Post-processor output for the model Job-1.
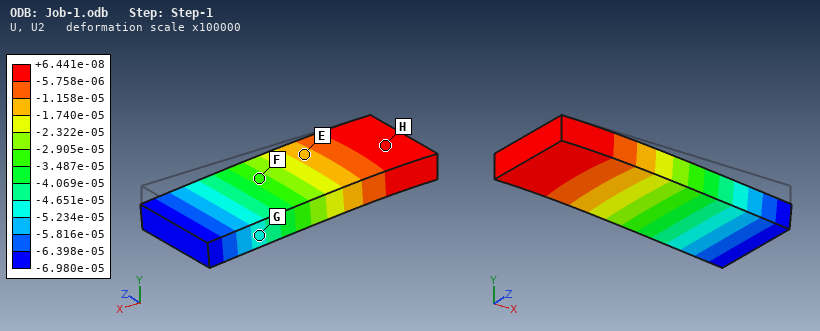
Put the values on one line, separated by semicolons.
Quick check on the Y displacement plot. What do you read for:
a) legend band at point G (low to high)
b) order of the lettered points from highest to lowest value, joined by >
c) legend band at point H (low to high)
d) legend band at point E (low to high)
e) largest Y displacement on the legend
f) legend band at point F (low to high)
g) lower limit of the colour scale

-5.234e-05 to -4.651e-05; H > E > F > G; -5.758e-06 to +6.441e-08; -1.740e-05 to -1.158e-05; +6.441e-08; -3.487e-05 to -2.905e-05; -6.980e-05
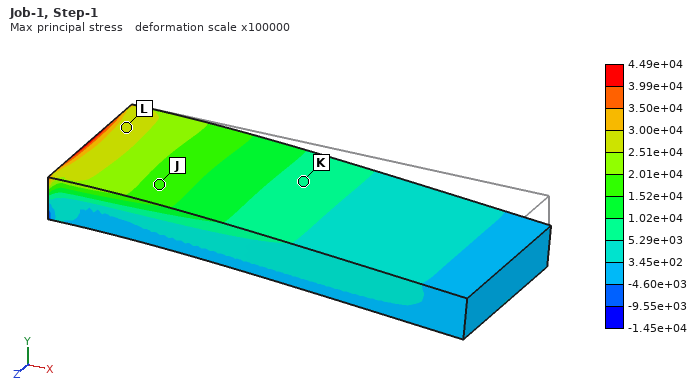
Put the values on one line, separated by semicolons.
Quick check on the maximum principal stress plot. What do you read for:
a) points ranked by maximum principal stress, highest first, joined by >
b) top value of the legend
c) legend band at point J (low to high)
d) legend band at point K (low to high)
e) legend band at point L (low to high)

L > J > K; 4.49e+04; 1.52e+04 to 2.01e+04; 5.29e+03 to 1.02e+04; 2.51e+04 to 3.00e+04
